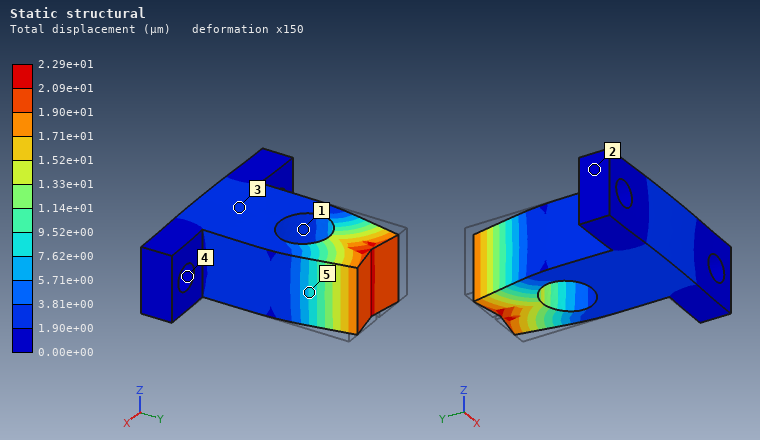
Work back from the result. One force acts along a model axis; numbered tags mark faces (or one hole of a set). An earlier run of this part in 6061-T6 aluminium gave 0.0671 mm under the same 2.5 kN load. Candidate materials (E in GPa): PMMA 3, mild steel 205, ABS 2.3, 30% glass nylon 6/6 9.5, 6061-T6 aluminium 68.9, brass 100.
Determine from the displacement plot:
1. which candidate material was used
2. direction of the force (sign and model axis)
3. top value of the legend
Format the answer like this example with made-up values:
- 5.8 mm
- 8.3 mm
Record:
- mild steel
- -Y
- 2.29e+01 µm
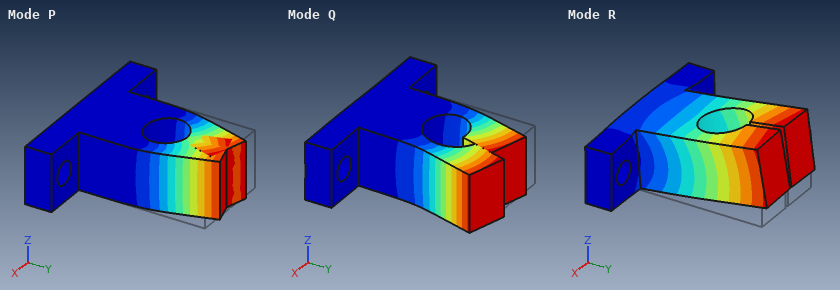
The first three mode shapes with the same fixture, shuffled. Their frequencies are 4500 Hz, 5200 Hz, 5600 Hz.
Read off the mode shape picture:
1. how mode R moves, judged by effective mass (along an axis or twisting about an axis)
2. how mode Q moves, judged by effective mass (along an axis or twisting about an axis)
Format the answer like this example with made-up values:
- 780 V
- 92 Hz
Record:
- along Z
- along X
